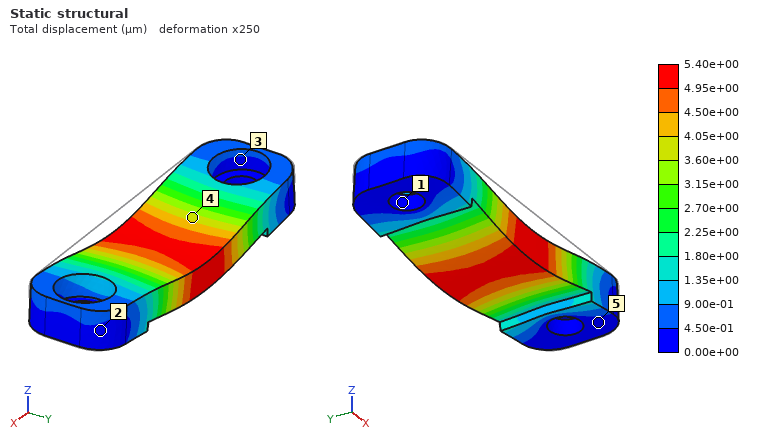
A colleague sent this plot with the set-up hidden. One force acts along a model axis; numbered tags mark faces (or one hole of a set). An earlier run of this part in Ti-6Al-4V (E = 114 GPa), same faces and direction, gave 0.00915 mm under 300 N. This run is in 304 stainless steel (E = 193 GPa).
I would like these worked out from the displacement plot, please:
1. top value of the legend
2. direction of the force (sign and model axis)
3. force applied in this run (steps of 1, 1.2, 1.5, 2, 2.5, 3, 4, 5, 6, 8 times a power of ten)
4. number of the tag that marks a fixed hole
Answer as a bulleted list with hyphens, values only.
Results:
- 5.40e+00 µm
- -Z
- 300 N
- 1
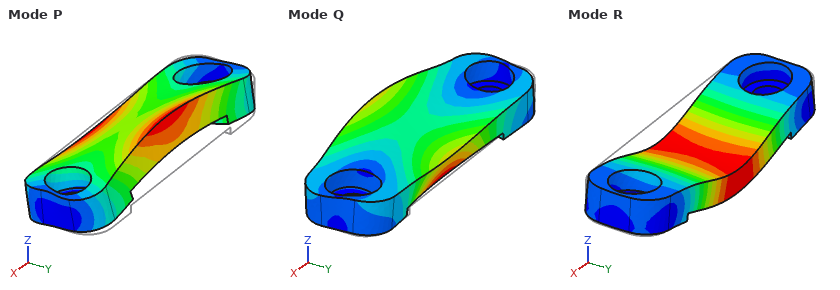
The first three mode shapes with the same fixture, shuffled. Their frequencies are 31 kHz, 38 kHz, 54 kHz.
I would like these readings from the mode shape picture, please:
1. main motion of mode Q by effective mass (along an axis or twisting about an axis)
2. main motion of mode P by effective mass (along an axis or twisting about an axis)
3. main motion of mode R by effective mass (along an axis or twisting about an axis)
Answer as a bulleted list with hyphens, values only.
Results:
- along Y
- along Y
- along Z
